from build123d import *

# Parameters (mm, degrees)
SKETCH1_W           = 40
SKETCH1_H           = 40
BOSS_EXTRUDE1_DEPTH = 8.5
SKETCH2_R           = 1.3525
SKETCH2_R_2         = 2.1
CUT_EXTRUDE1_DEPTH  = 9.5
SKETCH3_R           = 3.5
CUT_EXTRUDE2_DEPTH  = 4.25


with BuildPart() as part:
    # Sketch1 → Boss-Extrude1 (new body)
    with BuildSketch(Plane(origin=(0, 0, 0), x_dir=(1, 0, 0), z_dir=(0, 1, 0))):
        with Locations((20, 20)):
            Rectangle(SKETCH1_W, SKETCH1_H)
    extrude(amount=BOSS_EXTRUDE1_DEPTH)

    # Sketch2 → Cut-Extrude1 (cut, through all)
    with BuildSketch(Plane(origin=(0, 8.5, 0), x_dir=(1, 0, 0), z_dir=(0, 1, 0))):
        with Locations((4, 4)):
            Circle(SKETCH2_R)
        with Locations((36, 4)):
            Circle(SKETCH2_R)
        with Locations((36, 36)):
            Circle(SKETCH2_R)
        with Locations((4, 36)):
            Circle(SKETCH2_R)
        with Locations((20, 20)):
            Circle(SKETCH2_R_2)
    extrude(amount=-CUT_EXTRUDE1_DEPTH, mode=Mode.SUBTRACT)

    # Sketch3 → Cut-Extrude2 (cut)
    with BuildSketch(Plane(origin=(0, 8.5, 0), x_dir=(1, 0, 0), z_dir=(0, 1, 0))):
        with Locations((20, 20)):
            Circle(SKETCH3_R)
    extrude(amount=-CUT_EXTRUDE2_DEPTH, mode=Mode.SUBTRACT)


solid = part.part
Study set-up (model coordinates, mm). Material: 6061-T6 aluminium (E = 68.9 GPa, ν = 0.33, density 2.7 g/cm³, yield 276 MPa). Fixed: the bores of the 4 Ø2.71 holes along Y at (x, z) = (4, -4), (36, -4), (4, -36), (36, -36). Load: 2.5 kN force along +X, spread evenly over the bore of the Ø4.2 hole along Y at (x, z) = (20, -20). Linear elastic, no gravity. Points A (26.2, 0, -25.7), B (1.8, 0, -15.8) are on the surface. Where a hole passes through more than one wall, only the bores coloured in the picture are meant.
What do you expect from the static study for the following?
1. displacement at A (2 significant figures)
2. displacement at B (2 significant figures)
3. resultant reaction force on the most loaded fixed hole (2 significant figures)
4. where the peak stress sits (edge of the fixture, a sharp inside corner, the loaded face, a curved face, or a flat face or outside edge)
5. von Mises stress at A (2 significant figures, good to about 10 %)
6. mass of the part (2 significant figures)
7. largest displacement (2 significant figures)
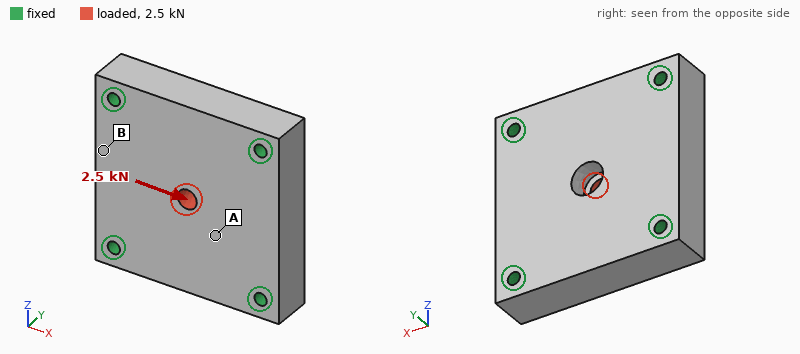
2.6 µm
2.4 µm
710 N
the loaded face
15 MPa
36 g
5.9 µm
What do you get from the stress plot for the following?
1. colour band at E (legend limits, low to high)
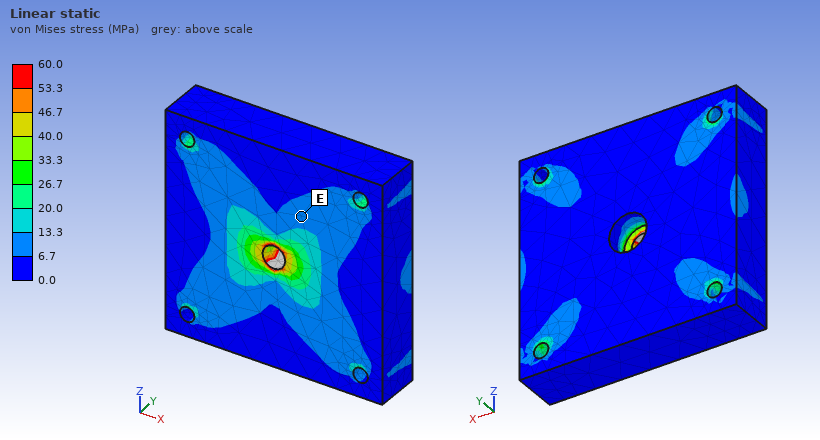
6.7 to 13.3 MPa
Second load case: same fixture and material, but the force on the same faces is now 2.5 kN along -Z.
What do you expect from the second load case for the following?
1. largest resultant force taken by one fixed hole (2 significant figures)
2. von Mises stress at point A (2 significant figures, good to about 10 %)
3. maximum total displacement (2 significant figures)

710 N
15 MPa
5.9 µm
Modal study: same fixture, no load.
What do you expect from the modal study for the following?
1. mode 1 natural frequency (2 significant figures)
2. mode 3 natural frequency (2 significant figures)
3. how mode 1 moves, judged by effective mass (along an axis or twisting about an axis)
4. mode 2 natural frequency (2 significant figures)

21 kHz
32 kHz
along Y
32 kHz
